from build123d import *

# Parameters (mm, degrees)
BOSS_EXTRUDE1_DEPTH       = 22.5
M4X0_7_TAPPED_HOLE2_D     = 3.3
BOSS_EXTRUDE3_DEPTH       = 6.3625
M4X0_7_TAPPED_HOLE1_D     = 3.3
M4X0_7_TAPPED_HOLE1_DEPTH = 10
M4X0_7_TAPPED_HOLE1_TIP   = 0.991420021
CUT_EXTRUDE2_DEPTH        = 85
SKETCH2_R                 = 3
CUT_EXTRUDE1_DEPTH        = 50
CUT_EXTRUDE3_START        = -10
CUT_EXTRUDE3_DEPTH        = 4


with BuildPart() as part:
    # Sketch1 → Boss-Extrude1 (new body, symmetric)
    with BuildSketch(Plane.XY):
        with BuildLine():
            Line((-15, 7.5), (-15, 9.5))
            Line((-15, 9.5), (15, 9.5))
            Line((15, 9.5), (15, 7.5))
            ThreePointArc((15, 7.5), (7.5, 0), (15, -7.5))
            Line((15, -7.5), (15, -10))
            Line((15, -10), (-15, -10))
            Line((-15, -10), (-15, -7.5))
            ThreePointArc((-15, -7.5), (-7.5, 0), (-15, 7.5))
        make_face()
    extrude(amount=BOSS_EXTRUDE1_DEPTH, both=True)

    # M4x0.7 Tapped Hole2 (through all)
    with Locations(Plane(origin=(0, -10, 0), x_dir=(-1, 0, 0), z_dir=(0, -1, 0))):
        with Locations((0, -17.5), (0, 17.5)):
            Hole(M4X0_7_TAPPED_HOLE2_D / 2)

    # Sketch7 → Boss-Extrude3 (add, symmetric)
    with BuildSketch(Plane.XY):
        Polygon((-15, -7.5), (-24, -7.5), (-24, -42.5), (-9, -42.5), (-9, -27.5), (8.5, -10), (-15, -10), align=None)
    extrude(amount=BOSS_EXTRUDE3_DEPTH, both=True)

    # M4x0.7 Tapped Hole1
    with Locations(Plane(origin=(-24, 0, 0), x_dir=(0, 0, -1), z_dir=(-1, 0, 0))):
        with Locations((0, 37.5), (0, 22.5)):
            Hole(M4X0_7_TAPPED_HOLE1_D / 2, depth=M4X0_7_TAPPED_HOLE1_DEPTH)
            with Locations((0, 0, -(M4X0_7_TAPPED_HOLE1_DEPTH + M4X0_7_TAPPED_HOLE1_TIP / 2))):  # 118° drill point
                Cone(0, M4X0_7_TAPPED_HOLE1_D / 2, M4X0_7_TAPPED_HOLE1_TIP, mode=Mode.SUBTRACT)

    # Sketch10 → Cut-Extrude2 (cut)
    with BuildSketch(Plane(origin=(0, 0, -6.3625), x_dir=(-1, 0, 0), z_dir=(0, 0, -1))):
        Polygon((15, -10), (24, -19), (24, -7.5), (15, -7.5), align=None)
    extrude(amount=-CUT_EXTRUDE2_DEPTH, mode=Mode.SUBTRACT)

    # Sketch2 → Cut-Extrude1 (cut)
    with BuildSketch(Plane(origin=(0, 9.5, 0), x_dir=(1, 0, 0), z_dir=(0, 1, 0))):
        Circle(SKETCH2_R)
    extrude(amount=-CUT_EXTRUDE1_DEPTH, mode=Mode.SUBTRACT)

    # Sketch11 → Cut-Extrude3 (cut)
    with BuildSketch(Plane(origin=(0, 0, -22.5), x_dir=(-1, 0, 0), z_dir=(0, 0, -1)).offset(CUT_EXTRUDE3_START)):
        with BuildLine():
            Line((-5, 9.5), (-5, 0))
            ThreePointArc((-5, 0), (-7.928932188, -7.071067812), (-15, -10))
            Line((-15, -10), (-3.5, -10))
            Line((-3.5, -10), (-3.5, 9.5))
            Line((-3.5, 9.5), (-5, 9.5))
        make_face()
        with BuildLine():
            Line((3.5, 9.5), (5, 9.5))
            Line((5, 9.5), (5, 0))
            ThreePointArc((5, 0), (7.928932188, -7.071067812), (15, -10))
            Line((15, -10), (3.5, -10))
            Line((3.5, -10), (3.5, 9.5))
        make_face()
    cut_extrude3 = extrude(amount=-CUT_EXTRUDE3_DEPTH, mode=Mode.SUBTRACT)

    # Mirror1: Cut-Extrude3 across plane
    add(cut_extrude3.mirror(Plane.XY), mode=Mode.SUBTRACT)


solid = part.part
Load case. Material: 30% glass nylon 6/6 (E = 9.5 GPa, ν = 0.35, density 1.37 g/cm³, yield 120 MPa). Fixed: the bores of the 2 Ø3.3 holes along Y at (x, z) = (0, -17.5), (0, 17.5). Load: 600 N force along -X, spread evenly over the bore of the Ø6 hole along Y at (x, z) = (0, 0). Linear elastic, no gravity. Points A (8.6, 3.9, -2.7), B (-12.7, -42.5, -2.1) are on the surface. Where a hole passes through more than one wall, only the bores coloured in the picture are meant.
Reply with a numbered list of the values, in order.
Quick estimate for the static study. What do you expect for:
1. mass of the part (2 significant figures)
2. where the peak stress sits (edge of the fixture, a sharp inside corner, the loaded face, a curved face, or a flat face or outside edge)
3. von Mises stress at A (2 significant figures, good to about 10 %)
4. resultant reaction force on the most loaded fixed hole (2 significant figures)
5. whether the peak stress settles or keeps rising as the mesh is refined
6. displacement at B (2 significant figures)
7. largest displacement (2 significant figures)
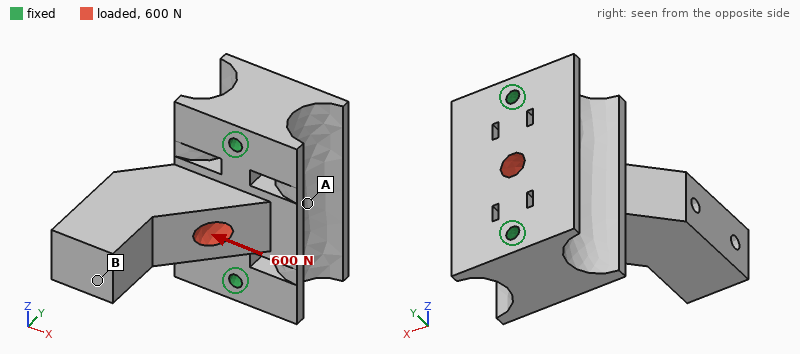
1. 33 g
2. edge of the fixture
3. 2.3 MPa
4. 300 N
5. keeps rising
6. 41 µm
7. 44 µm
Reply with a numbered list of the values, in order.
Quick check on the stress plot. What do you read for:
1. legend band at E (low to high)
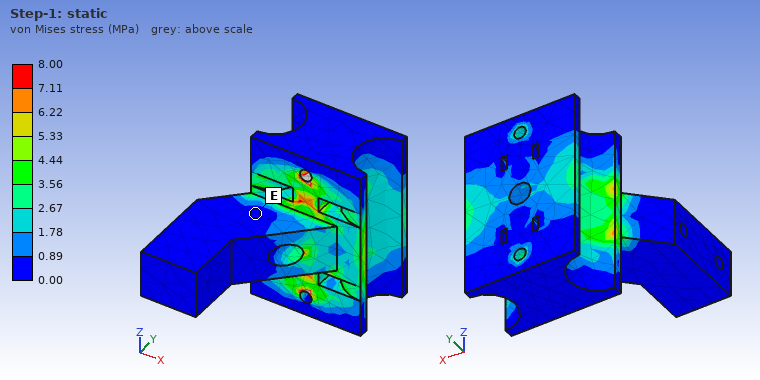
1. 0.00 to 0.89 MPa
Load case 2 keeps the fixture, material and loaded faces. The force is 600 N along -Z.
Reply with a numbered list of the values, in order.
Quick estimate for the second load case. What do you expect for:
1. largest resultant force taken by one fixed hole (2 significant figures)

1. 310 N
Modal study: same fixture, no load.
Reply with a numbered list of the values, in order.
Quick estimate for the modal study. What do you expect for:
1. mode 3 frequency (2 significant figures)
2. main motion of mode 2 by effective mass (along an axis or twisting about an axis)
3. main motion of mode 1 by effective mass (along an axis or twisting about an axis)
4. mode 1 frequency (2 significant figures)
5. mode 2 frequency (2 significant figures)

1. 9300 Hz
2. along Z
3. along X
4. 2700 Hz
5. 3300 Hz
